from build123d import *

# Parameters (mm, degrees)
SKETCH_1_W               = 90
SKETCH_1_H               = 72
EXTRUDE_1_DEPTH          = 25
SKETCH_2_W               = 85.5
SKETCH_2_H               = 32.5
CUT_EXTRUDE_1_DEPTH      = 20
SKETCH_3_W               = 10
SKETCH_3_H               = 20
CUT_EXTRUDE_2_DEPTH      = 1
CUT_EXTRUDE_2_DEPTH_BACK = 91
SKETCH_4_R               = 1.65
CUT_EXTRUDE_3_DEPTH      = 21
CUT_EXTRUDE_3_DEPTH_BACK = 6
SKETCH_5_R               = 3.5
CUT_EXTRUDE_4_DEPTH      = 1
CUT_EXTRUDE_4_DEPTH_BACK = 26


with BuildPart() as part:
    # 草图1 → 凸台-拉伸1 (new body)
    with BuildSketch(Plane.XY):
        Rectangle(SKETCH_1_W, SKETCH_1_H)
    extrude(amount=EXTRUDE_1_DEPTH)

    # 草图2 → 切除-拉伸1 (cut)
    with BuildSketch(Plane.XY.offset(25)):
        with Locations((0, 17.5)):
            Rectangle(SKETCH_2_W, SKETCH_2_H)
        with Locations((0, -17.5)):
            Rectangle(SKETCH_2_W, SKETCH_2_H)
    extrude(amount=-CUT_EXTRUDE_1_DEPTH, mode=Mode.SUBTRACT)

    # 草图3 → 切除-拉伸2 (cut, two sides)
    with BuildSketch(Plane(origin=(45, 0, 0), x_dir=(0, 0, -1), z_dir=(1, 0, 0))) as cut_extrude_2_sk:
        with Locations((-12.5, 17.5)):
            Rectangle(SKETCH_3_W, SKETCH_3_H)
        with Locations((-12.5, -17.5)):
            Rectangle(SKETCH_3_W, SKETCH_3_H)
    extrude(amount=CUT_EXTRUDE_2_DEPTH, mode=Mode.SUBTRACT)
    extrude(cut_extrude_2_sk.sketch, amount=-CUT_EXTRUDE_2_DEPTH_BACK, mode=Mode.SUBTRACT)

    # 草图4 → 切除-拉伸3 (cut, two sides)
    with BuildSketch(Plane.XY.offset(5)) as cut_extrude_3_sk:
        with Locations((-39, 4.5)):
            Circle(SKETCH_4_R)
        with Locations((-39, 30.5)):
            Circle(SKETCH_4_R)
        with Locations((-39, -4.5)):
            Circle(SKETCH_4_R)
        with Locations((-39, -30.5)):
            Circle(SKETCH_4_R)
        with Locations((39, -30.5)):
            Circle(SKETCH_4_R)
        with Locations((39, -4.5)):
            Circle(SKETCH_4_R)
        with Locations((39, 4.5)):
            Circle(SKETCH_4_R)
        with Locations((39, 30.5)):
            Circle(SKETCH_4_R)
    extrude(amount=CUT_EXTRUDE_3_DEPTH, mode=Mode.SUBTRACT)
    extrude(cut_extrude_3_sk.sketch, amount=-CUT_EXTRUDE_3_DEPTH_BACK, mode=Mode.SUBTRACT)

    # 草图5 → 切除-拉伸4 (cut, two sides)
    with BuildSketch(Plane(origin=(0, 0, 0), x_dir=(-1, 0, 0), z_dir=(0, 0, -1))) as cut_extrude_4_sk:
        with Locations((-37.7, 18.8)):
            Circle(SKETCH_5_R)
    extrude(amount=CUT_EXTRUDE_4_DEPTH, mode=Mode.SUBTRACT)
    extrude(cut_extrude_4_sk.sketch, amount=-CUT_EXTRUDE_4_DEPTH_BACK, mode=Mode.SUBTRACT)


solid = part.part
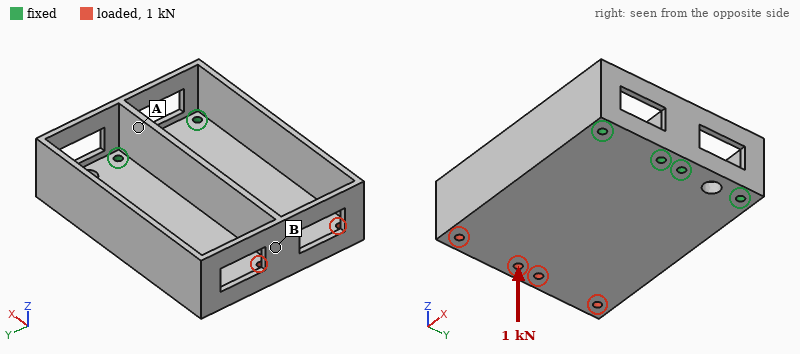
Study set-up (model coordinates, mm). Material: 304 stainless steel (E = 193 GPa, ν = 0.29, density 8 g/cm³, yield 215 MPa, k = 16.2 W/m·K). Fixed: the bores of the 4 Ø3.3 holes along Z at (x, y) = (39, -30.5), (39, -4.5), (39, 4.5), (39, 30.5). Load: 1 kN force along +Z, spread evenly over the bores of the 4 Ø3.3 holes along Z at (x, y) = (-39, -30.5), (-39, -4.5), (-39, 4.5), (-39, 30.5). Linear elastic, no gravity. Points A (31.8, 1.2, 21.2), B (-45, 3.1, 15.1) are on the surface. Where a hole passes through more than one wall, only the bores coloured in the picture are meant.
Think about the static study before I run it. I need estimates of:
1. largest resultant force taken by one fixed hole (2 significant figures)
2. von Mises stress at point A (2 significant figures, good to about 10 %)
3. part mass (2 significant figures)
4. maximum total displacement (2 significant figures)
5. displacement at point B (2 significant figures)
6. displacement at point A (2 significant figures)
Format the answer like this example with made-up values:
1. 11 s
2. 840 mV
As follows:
1. 420 N
2. 52 MPa
3. 390 g
4. 0.24 mm
5. 0.23 mm
6. 0.044 mm
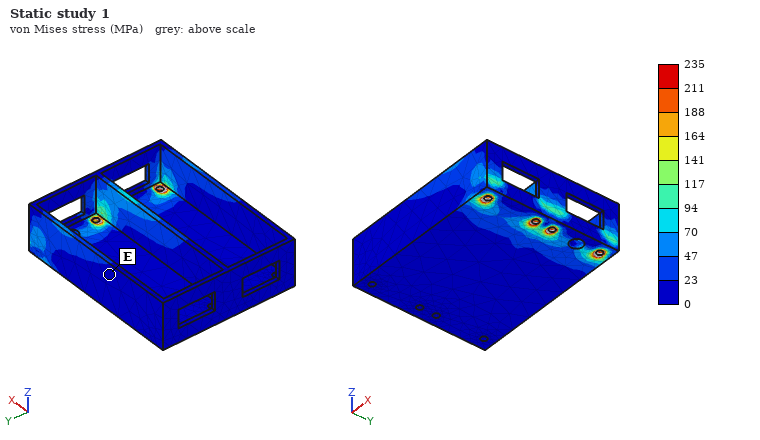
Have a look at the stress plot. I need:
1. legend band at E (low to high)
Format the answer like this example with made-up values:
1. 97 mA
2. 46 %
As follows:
1. 0 to 23 MPa
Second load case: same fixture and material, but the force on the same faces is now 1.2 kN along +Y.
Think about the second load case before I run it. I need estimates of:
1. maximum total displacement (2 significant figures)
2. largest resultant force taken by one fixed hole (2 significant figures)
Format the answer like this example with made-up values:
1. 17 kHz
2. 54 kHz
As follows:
1. 15 µm
2. 1.5 kN
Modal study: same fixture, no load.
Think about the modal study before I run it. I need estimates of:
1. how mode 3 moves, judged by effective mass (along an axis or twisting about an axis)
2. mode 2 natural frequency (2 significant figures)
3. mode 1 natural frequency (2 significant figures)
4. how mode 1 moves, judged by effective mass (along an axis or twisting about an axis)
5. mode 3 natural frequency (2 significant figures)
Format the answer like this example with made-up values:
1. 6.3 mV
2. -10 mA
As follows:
1. along Y
2. 1300 Hz
3. 910 Hz
4. along Z
5. 4100 Hz
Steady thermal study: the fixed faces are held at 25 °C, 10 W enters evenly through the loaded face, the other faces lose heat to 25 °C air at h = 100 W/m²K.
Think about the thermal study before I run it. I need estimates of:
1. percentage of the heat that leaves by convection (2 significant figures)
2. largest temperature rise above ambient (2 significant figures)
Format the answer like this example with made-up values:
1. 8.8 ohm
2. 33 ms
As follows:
1. 99 %
2. 23 K
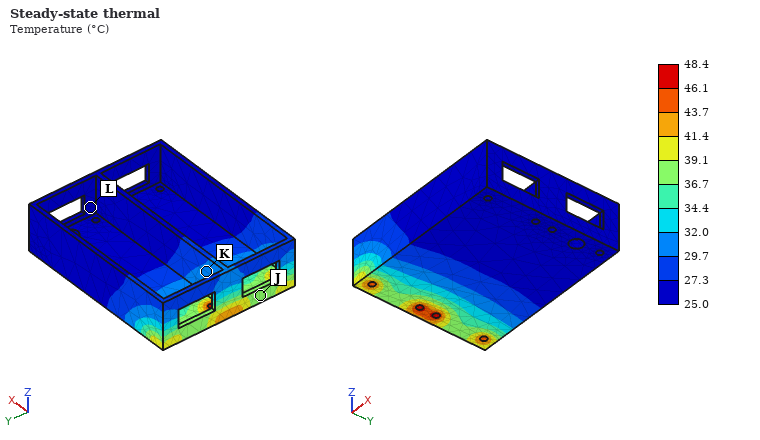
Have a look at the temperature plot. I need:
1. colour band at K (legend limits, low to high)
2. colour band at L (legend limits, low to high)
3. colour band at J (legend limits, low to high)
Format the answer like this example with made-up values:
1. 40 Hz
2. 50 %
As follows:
1. 29.7 to 32.0 °C
2. 25.0 to 27.3 °C
3. 36.7 to 39.1 °C
